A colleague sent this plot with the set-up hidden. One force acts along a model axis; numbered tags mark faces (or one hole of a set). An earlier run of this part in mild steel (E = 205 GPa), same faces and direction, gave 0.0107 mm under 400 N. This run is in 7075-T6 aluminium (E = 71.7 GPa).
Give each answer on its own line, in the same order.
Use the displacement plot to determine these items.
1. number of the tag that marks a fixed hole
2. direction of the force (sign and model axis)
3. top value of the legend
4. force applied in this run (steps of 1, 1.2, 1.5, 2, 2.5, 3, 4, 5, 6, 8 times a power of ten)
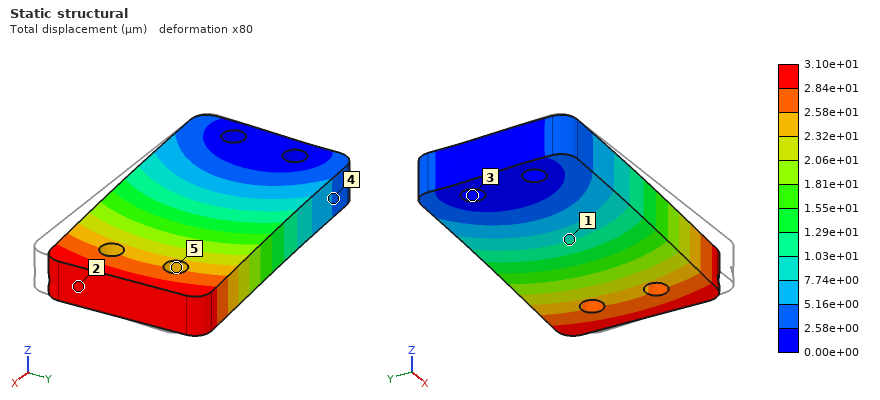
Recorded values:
3
+Y
3.10e+01 µm
400 N
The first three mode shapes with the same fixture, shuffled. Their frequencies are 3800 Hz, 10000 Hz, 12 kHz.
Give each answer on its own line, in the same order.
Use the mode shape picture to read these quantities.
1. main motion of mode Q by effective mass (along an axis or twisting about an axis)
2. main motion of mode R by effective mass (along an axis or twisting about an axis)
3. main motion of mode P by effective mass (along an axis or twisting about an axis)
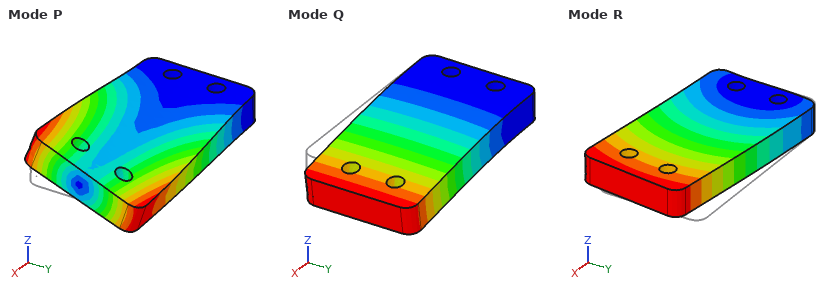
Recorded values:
along Z
along Y
twisting about X
